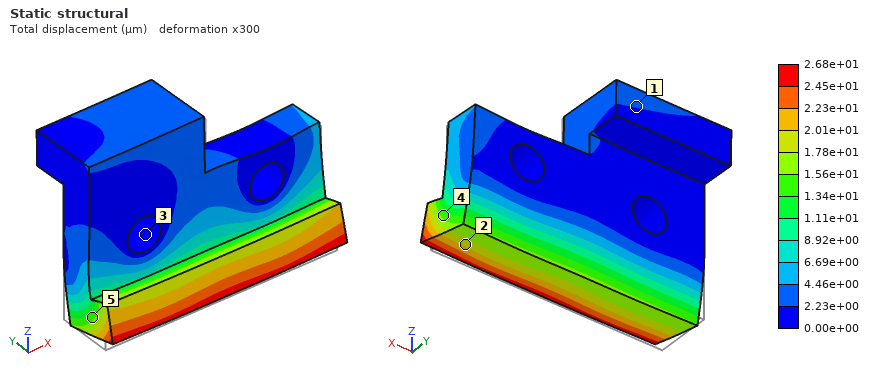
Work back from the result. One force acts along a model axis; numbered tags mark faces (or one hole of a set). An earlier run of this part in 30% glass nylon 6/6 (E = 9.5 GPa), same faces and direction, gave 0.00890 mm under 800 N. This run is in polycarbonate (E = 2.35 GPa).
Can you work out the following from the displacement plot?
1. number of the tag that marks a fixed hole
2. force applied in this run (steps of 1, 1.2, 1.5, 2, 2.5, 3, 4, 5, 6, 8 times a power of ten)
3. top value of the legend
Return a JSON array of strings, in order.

["3", "600 N", "2.68e+01 µm"]
